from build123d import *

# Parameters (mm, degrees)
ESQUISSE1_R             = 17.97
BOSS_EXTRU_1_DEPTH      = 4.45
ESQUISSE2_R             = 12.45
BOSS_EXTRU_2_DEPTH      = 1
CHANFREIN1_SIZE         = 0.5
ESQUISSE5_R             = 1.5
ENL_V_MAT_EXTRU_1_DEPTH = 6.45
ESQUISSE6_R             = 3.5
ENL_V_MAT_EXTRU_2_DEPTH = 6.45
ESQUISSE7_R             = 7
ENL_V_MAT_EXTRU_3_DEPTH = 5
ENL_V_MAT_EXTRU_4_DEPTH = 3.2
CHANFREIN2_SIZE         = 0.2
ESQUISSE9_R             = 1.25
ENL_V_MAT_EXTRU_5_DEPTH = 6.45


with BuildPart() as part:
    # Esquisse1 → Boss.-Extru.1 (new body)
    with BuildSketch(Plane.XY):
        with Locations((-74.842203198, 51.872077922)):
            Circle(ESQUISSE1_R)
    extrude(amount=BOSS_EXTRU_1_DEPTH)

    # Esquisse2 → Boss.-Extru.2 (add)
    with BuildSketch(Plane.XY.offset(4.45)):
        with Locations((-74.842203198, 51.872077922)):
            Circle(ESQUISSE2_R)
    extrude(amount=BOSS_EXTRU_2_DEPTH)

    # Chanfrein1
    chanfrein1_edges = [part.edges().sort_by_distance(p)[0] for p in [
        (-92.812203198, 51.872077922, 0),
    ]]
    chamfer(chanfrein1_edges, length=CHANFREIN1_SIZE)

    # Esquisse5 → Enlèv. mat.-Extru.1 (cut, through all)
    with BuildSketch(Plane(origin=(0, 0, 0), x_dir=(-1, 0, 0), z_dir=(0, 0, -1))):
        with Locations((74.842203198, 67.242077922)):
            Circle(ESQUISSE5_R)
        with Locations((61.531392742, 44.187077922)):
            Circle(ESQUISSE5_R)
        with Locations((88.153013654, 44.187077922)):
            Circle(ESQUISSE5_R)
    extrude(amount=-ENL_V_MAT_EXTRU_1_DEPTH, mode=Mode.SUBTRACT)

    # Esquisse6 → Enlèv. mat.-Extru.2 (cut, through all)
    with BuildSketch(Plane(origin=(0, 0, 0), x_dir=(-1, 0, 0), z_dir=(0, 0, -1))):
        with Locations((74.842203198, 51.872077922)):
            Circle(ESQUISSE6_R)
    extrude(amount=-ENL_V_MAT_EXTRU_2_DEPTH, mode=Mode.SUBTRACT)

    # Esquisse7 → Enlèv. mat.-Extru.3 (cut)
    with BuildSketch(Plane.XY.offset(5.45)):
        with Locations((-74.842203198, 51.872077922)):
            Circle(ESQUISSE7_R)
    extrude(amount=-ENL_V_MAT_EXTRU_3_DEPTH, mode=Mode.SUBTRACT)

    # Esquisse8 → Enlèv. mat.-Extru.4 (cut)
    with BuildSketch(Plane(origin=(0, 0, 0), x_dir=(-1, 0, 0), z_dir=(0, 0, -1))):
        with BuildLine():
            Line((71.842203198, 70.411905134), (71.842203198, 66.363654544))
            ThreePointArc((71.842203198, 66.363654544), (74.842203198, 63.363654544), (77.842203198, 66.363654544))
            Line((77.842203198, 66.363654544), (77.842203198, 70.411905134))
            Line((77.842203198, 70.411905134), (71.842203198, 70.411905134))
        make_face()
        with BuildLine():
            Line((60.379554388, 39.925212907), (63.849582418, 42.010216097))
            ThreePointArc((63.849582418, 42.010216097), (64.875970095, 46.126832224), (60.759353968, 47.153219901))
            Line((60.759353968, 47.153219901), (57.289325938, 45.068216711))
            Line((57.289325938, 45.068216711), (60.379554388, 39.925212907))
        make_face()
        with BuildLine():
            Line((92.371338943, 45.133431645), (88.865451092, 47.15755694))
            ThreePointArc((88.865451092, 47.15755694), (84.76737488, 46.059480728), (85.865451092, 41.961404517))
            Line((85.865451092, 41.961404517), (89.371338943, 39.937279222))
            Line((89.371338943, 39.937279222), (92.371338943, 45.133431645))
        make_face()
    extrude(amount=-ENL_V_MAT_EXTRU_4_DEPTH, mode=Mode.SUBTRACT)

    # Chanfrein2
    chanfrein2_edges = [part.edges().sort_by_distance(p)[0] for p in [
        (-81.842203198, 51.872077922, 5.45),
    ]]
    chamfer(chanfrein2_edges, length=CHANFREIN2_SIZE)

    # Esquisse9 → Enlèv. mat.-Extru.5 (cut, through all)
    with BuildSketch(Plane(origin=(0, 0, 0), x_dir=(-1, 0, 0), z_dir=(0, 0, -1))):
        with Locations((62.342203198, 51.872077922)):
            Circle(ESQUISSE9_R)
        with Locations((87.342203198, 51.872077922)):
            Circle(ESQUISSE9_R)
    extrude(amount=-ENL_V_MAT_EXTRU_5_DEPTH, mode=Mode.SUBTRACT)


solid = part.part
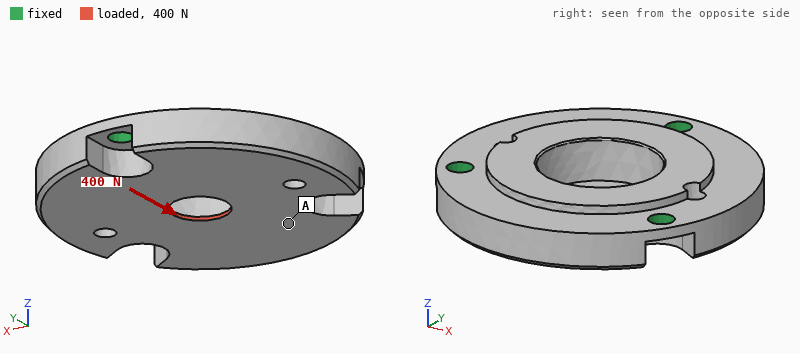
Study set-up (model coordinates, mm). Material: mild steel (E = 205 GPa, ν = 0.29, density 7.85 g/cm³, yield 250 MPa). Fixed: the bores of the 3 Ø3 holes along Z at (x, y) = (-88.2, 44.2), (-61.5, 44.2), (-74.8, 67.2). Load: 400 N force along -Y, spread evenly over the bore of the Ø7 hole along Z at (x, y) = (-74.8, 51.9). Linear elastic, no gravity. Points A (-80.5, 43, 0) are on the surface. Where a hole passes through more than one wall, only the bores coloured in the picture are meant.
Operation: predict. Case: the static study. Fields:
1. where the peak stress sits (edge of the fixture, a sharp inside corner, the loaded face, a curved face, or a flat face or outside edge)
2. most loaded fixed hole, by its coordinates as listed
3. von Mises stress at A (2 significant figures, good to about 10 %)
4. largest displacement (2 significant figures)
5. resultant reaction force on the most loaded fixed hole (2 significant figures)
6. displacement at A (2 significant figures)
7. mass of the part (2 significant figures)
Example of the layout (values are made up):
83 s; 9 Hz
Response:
the loaded face; (-74.8, 67.2); 7.6 MPa; 2.0 µm; 170 N; 0.96 µm; 30 g
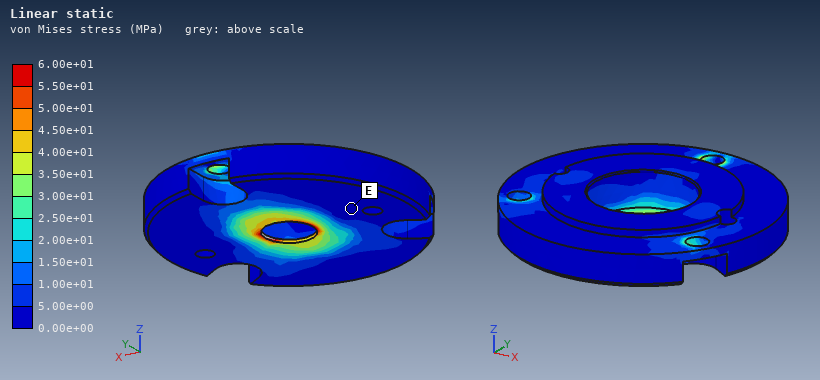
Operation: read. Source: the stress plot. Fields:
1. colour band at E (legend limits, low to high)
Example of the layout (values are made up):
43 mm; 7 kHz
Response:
0.00e+00 to 5.00e+00 MPa
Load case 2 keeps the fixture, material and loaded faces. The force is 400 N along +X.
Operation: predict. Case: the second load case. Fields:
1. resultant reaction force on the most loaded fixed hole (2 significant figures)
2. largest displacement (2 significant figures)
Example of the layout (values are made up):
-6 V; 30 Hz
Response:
150 N; 1.8 µm
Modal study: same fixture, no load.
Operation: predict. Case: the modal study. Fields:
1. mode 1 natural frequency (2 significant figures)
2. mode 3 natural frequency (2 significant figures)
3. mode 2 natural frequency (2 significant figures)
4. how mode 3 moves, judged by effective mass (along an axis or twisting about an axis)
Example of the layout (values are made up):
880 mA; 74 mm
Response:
13 kHz; 16 kHz; 13 kHz; along Z
